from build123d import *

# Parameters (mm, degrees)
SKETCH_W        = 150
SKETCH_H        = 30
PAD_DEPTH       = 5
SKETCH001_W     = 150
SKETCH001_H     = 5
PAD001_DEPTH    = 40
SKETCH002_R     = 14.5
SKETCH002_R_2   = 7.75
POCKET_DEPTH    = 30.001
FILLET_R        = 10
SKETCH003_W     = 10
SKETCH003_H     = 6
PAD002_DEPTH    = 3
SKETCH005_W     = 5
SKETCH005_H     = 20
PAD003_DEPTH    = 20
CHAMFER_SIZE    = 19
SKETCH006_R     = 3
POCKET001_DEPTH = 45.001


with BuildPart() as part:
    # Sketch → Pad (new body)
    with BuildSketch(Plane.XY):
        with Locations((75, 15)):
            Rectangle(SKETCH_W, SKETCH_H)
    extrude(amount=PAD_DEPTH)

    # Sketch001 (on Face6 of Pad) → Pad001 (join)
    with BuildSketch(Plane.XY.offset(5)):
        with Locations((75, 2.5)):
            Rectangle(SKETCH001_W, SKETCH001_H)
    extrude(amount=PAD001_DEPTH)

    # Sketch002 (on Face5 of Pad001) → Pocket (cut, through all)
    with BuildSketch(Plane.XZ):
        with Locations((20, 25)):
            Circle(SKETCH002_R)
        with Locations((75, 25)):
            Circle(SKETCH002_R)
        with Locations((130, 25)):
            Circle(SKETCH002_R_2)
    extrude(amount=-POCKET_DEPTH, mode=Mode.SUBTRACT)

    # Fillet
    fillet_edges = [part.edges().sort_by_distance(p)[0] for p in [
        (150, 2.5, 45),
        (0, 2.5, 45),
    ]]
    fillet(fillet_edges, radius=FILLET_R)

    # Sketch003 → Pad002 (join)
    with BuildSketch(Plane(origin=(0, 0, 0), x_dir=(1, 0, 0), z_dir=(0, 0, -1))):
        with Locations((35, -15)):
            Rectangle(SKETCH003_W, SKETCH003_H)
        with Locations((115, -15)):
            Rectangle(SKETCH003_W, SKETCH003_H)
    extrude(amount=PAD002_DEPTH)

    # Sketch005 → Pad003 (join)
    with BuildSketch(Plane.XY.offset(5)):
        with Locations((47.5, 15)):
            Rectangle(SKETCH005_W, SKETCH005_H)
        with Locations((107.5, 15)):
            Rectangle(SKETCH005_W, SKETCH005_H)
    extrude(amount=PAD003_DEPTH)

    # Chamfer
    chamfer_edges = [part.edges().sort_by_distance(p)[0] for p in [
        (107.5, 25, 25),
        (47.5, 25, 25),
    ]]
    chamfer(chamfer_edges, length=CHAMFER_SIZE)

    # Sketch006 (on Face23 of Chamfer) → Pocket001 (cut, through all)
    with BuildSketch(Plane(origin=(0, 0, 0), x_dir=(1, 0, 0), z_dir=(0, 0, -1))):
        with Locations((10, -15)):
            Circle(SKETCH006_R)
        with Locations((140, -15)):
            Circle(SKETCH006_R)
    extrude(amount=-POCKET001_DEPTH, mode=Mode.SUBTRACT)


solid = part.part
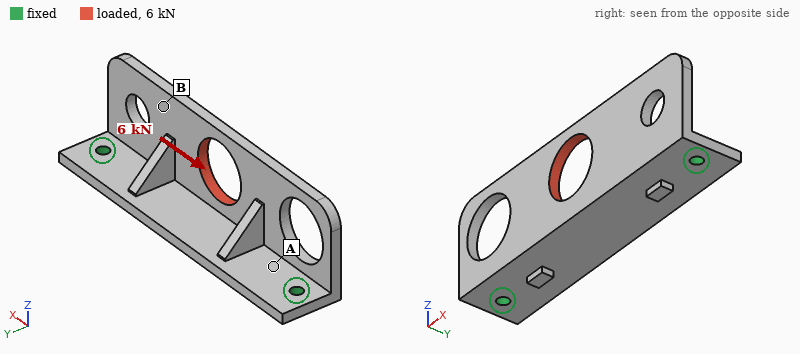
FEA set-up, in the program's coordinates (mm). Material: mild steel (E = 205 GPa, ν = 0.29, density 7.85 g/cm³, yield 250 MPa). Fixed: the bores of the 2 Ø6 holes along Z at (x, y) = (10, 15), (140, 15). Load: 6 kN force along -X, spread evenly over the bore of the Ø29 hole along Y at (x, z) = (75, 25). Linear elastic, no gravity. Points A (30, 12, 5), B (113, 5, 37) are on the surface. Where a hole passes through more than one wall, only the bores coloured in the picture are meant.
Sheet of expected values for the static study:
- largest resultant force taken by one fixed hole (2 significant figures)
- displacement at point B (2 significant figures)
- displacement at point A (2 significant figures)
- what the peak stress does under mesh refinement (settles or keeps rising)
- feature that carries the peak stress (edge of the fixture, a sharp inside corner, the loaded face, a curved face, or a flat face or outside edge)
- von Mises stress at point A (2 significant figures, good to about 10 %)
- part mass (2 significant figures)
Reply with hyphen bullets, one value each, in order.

- 3.2 kN
- 20 µm
- 5.9 µm
- keeps rising
- edge of the fixture
- 33 MPa
- 370 g
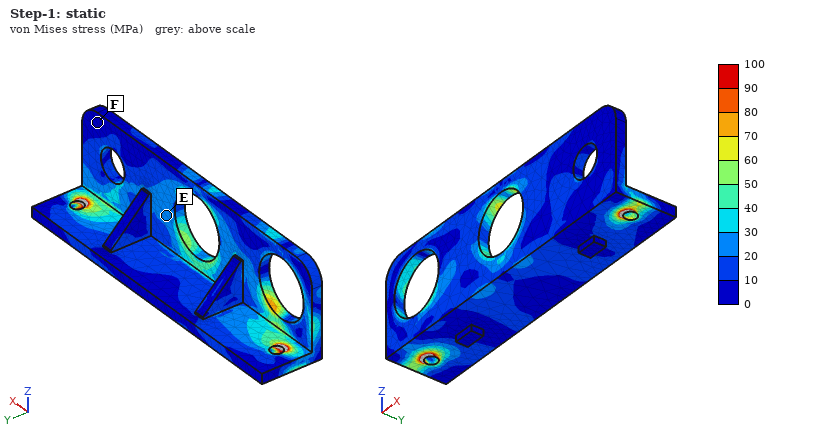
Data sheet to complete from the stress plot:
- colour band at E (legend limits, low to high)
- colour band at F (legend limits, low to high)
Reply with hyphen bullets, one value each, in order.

- 20 to 30 MPa
- 0 to 10 MPa
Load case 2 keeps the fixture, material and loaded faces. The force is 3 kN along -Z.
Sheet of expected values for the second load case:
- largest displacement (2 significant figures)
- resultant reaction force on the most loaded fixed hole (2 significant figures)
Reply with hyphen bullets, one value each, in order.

- 91 µm
- 1.8 kN
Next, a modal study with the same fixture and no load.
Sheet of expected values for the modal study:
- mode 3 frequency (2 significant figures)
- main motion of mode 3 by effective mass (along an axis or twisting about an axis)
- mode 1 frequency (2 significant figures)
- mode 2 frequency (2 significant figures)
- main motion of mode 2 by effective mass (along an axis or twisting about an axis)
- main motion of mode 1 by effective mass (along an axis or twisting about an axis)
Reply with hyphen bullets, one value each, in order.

- 3000 Hz
- along Z
- 1300 Hz
- 2200 Hz
- twisting about Z
- along Y
